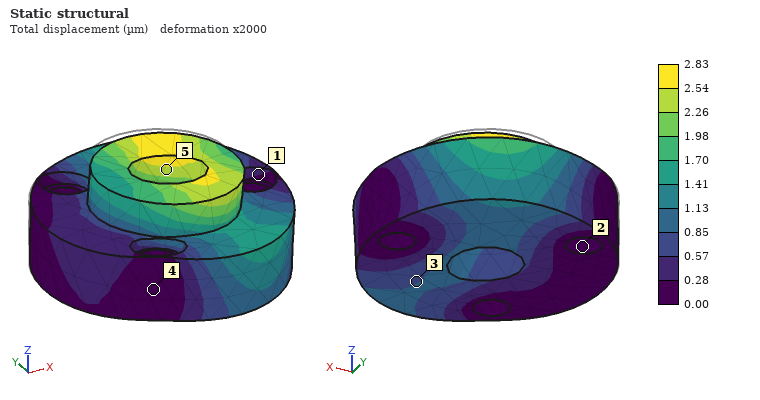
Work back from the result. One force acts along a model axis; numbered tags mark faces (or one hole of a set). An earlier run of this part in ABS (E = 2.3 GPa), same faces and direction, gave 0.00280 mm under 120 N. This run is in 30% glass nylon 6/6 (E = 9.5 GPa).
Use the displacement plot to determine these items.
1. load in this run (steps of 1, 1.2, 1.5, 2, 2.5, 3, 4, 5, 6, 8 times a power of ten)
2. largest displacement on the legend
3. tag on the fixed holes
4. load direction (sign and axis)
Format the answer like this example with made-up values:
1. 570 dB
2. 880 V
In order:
1. 500 N
2. 2.83 µm
3. 2
4. -Y
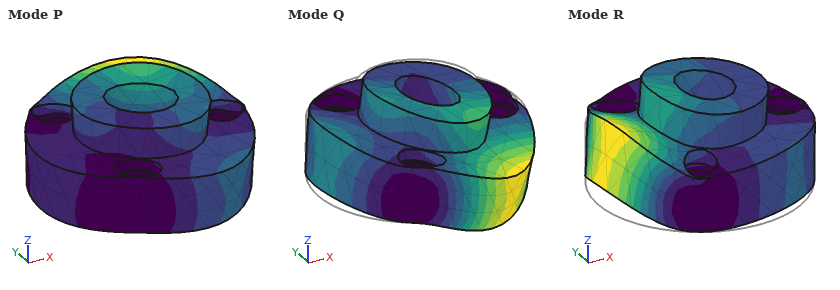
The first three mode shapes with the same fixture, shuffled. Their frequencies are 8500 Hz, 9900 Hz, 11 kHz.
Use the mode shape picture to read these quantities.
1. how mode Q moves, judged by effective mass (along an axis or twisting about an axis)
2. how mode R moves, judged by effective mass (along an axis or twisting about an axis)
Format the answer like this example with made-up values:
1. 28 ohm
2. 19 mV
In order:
1. along Z
2. along Z
